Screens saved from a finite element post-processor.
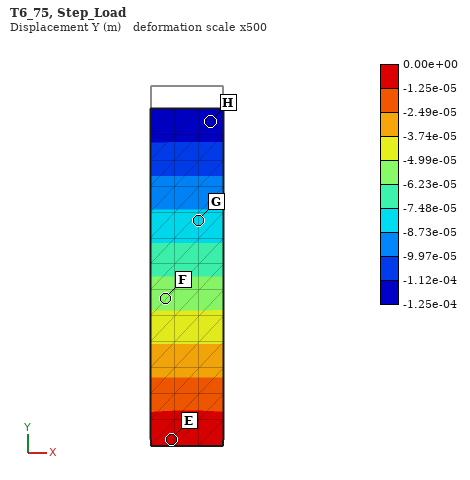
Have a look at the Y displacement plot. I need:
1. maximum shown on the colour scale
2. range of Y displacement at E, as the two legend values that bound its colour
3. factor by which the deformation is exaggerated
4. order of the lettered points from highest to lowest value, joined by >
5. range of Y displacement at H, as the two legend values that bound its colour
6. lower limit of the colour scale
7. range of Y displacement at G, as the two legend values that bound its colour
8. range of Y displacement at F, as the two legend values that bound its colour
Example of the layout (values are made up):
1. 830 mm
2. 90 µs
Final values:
1. 0.00e+00 m
2. -1.25e-05 to 0.00e+00 m
3. 500
4. E > F > G > H
5. -1.25e-04 to -1.12e-04 m
6. -1.25e-04 m
7. -8.73e-05 to -7.48e-05 m
8. -6.23e-05 to -4.99e-05 m
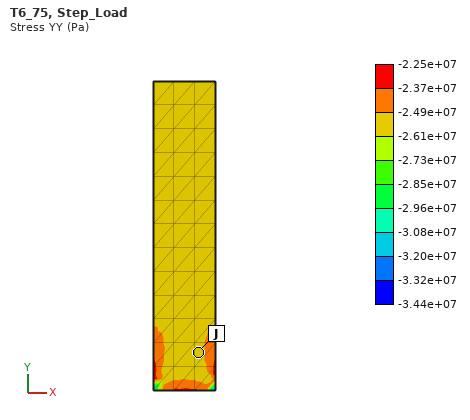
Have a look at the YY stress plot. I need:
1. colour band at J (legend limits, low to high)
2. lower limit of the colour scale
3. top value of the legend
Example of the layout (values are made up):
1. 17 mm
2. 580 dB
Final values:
1. -2.61e+07 to -2.49e+07 Pa
2. -3.44e+07 Pa
3. -2.25e+07 Pa
